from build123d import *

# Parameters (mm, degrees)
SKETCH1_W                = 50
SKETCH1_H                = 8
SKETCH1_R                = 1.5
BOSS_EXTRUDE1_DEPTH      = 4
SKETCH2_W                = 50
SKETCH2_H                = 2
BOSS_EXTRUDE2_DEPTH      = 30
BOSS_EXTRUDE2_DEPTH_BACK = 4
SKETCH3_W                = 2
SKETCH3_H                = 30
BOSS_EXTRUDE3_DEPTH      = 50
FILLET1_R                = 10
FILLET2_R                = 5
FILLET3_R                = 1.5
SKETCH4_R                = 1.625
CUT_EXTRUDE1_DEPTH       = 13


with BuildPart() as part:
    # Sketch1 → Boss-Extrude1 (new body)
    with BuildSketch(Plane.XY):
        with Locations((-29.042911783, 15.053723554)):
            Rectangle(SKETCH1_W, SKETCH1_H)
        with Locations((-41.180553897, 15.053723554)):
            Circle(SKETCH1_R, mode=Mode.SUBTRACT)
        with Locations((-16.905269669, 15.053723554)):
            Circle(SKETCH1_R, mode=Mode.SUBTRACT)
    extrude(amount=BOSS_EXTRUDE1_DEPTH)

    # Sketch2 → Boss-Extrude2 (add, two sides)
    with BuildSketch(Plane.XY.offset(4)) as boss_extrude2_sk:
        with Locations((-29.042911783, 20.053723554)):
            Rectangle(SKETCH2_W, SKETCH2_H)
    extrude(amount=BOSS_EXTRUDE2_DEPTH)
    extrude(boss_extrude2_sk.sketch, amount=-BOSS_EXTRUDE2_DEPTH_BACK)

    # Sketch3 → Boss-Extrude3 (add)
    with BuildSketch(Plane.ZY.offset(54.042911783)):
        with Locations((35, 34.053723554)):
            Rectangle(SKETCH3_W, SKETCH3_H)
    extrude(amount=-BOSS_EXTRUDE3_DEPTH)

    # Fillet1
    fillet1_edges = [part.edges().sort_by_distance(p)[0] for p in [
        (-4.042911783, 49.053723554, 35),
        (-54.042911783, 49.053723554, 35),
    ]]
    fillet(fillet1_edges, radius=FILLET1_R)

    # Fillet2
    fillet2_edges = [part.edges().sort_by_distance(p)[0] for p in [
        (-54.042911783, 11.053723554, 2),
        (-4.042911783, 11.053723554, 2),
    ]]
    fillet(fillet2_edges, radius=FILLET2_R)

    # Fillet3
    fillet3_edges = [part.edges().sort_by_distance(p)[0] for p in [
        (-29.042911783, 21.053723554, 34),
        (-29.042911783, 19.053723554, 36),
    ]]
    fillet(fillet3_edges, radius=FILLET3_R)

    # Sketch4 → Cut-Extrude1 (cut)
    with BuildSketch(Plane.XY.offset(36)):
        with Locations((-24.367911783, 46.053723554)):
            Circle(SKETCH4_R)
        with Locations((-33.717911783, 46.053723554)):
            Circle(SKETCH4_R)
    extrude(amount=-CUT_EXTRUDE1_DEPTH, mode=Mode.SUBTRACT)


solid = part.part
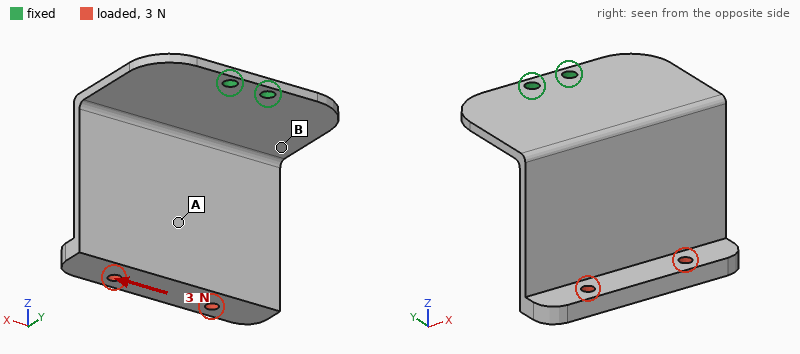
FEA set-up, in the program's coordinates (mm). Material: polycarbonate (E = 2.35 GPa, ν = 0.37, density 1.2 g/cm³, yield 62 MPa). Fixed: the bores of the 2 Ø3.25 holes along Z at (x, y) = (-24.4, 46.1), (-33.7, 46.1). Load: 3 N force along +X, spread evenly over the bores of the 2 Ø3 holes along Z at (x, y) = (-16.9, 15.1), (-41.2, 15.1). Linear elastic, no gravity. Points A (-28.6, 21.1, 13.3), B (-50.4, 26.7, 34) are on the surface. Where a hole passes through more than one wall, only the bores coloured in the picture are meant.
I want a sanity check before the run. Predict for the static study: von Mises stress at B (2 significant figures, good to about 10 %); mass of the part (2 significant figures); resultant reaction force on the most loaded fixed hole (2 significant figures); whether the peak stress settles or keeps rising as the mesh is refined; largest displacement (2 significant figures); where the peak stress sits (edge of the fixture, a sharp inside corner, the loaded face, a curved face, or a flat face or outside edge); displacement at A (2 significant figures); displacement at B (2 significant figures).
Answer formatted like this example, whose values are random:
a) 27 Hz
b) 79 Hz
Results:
a) 1.3 MPa
b) 9.3 g
c) 9.5 N
d) keeps rising
e) 0.75 mm
f) edge of the fixture
g) 0.38 mm
h) 0.31 mm
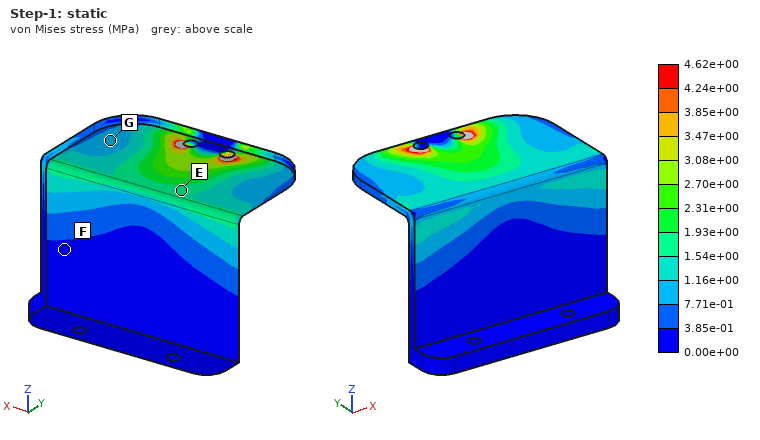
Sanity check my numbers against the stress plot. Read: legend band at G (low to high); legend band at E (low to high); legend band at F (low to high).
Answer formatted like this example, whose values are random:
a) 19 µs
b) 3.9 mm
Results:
a) 7.71e-01 to 1.16e+00 MPa
b) 1.54e+00 to 1.93e+00 MPa
c) 0.00e+00 to 3.85e-01 MPa
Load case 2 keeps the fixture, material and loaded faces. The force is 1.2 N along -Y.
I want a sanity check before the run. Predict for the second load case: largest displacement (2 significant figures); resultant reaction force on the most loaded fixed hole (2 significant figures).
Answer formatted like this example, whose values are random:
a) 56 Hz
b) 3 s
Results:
a) 0.75 mm
b) 0.60 N
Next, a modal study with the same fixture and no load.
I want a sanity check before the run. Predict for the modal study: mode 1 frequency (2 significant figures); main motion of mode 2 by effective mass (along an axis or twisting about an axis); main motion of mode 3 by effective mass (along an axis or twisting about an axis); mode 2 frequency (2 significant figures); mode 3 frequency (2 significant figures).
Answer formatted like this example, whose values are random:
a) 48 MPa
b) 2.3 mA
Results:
a) 110 Hz
b) along X
c) along Z
d) 170 Hz
e) 360 Hz
